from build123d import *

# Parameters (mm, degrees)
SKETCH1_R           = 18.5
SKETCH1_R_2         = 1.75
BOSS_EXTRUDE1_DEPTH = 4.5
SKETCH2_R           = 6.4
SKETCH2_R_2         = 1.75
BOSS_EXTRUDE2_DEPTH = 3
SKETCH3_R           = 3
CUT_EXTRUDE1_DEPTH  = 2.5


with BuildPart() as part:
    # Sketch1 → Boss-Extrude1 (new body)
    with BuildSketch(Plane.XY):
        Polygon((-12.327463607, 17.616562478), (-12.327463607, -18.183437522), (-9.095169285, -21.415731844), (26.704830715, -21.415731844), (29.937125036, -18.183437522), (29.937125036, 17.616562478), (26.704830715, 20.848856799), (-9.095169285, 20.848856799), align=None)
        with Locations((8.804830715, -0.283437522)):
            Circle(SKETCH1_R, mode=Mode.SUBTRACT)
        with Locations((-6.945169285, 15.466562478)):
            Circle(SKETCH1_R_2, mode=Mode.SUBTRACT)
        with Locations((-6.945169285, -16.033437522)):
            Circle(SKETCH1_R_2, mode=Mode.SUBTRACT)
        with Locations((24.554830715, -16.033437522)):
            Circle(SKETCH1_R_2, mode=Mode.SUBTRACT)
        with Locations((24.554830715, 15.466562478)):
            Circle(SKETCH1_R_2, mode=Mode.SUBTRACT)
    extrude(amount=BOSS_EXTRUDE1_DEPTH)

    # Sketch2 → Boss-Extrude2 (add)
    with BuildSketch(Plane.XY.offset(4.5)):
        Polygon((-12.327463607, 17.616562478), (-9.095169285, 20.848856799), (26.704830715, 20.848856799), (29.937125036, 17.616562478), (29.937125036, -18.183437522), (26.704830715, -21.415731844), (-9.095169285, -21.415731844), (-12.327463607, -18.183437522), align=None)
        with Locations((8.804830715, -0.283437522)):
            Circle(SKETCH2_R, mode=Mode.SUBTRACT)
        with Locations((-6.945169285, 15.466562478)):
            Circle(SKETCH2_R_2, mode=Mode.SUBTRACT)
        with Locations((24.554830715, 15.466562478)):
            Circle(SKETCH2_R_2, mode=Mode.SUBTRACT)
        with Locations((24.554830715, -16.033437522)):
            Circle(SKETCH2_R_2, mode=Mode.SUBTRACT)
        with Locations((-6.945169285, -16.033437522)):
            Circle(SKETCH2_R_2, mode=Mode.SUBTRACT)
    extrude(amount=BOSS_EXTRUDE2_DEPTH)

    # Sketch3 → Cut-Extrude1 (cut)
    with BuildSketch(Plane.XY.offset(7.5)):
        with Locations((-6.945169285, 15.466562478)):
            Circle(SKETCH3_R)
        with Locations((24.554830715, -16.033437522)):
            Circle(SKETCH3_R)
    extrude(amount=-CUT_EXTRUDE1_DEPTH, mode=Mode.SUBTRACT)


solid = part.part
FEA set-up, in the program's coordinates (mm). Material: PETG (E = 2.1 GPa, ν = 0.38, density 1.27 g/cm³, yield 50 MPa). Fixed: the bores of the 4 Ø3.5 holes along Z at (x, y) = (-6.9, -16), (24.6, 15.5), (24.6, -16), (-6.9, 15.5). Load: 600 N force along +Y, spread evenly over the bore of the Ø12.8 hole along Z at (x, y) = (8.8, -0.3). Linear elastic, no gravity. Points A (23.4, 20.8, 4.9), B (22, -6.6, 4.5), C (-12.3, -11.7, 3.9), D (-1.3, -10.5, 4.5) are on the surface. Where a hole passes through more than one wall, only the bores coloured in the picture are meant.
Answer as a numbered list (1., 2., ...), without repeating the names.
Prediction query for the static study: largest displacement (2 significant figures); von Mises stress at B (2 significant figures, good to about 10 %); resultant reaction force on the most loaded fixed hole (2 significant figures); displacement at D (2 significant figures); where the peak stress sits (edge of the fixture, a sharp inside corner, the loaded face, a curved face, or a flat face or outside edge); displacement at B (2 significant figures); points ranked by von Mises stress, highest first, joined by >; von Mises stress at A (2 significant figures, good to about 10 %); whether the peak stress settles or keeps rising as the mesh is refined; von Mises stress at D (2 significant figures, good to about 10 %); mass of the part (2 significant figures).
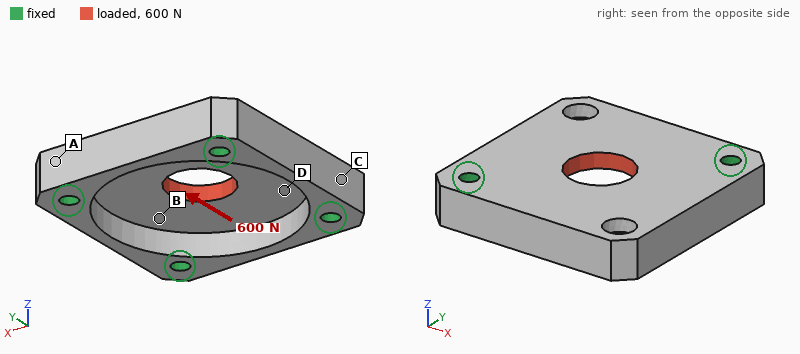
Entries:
1. 60 µm
2. 4.1 MPa
3. 180 N
4. 23 µm
5. edge of the fixture
6. 24 µm
7. D > B > A > C
8. 2.6 MPa
9. keeps rising
10. 5.5 MPa
11. 9.7 g
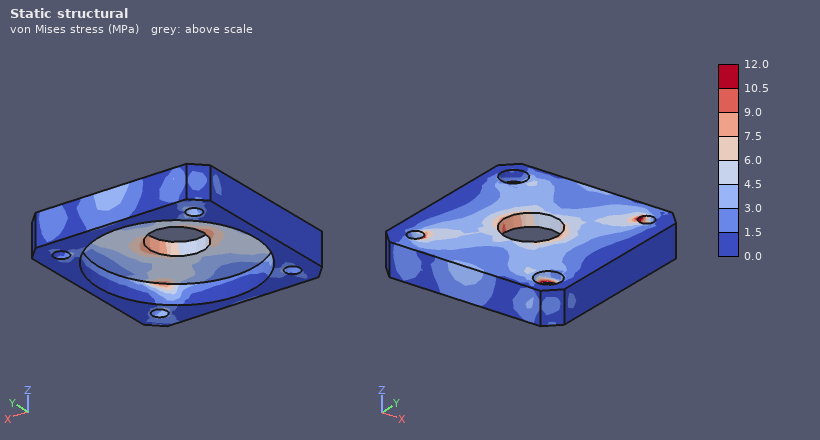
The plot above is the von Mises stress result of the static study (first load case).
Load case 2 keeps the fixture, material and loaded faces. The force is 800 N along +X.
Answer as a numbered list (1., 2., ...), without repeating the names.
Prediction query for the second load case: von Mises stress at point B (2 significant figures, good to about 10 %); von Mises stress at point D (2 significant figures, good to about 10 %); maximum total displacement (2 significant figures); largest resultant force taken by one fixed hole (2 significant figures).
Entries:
1. 6.3 MPa
2. 7.3 MPa
3. 80 µm
4. 240 N
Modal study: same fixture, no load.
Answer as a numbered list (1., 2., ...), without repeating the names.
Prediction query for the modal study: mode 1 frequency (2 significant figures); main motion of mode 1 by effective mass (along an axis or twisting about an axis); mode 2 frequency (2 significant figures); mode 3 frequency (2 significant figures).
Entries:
1. 4300 Hz
2. along Z
3. 6200 Hz
4. 6600 Hz
